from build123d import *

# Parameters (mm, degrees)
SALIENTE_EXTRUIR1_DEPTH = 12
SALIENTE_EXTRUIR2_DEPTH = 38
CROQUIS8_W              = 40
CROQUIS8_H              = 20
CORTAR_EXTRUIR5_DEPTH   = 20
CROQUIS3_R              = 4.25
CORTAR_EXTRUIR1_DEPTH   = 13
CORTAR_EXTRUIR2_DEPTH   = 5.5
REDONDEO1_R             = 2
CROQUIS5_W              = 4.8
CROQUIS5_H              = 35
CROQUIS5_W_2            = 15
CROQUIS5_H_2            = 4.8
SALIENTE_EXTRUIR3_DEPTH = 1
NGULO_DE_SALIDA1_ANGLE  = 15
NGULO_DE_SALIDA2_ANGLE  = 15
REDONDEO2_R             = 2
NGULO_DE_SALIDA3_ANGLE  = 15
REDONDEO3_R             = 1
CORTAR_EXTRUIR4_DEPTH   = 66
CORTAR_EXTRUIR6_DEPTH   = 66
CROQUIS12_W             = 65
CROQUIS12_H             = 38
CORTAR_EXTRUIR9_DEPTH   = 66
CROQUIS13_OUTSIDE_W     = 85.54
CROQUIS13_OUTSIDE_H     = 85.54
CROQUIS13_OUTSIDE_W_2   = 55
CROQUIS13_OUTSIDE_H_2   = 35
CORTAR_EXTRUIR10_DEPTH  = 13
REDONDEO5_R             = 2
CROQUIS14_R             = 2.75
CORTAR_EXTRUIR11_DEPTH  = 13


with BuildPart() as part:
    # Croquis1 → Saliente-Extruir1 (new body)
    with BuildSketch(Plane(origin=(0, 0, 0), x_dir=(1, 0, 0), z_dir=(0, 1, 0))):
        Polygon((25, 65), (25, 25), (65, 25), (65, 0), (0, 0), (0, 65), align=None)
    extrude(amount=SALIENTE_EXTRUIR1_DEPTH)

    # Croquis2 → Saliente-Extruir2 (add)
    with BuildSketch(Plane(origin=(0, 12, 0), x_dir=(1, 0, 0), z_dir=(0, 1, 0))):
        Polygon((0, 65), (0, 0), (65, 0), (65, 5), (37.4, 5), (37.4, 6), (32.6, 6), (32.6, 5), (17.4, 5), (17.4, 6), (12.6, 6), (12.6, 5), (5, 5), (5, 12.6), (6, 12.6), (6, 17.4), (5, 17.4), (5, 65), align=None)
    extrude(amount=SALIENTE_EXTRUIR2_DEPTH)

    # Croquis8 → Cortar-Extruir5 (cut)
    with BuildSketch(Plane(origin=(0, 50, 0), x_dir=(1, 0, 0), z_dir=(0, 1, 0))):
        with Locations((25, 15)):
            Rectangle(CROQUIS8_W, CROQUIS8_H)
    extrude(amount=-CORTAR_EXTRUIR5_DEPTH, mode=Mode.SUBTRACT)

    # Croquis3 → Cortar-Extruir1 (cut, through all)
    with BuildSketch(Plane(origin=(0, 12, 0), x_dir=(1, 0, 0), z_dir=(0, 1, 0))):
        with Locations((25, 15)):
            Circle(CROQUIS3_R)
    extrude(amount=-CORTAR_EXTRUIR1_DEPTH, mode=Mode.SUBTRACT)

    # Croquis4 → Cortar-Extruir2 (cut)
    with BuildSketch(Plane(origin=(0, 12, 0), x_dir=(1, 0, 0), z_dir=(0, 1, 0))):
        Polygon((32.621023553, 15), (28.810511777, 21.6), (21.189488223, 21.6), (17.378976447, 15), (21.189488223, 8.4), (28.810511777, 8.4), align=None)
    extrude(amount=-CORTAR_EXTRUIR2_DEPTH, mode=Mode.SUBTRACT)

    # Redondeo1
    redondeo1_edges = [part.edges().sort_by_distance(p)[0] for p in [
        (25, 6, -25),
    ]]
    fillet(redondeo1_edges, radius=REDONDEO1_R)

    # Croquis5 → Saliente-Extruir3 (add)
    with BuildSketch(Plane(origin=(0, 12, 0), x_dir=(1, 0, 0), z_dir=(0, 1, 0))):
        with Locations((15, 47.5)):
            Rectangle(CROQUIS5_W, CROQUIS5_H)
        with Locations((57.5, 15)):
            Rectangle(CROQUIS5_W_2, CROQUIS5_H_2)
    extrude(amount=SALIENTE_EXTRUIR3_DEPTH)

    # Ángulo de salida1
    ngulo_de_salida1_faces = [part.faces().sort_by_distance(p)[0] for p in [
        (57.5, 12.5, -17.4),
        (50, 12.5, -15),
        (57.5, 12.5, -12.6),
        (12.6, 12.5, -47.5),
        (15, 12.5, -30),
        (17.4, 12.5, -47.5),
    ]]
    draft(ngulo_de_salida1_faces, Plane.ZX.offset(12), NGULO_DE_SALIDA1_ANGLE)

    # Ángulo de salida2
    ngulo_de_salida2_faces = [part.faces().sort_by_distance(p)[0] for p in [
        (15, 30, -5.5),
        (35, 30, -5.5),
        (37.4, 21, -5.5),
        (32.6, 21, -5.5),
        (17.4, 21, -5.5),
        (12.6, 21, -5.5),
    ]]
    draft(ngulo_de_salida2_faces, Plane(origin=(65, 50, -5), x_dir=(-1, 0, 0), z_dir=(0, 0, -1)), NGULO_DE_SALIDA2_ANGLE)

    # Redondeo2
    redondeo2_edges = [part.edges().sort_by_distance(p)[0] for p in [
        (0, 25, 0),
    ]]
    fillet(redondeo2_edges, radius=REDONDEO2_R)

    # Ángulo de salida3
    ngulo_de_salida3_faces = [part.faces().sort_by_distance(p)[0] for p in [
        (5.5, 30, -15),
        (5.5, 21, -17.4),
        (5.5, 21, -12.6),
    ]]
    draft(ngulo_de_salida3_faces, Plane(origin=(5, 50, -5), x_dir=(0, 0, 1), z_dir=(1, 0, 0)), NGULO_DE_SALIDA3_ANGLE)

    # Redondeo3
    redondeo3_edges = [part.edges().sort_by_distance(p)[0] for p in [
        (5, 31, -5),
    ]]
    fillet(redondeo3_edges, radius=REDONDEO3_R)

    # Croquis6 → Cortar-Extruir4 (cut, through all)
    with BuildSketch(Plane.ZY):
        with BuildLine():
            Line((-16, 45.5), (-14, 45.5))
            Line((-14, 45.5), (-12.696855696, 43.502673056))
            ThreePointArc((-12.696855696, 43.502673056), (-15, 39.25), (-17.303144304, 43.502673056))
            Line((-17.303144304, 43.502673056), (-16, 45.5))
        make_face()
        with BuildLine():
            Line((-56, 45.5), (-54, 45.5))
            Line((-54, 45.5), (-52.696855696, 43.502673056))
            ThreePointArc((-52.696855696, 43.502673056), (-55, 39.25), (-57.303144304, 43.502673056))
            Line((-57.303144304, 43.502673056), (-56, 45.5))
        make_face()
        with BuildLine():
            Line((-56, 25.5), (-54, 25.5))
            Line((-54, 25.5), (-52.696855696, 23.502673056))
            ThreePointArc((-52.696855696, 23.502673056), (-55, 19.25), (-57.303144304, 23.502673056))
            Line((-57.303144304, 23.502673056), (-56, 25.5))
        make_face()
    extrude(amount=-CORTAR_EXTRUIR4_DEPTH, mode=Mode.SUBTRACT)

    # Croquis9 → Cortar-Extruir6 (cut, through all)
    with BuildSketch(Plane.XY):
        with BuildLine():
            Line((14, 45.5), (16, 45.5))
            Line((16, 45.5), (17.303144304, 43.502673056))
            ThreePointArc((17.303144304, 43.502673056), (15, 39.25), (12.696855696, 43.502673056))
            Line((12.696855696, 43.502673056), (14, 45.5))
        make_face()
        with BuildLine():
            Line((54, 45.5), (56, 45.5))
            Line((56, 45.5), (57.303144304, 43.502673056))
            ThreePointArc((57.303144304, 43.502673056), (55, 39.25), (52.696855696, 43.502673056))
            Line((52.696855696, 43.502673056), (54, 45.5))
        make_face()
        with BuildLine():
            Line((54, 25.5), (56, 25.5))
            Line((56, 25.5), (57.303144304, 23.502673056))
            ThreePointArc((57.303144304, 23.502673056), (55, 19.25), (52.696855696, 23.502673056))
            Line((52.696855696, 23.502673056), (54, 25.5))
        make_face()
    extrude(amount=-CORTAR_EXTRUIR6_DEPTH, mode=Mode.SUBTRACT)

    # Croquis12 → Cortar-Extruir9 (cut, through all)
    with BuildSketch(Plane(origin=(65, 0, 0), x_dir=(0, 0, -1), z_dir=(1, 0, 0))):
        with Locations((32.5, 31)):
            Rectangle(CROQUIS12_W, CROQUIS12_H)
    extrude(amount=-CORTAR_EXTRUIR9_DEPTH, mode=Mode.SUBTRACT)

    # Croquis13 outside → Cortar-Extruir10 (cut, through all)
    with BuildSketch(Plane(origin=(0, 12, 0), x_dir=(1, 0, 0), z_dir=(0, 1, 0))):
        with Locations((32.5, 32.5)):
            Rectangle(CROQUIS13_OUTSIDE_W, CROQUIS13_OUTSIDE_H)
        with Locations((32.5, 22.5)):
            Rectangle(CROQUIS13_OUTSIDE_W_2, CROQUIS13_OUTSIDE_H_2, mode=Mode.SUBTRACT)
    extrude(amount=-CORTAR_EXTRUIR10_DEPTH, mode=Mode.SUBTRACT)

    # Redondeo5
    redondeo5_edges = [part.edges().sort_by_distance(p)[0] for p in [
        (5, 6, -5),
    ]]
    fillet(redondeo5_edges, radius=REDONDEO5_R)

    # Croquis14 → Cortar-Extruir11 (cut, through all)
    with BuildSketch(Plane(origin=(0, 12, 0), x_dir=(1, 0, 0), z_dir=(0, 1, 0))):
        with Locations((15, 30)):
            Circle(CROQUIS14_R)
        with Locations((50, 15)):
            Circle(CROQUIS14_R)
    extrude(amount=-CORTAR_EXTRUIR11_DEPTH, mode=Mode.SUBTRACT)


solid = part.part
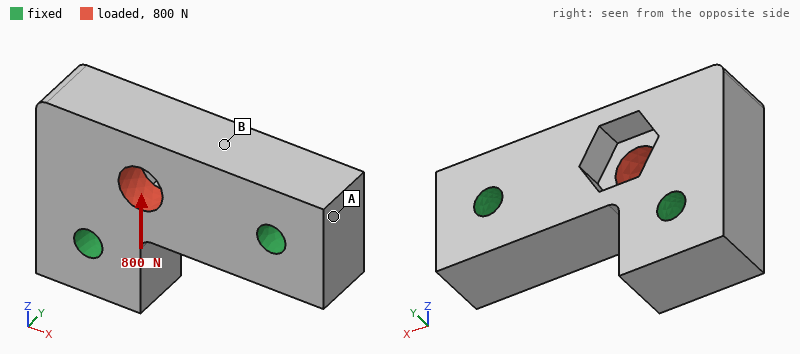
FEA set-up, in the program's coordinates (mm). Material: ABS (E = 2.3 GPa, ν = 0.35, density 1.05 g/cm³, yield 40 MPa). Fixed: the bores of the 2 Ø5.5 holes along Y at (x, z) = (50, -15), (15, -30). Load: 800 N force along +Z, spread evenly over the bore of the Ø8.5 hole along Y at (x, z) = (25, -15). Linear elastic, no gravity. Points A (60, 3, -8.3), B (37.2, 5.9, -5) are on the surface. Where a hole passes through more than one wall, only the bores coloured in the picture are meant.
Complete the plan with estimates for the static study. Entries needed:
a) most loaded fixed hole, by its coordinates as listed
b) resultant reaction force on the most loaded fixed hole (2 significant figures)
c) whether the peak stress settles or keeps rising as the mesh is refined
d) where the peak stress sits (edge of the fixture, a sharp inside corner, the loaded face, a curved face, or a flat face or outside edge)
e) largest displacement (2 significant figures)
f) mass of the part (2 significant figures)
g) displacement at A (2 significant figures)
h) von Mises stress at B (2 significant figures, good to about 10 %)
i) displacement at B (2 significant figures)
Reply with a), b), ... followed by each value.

a) (15, -30)
b) 630 N
c) keeps rising
d) edge of the fixture
e) 88 µm
f) 16 g
g) 14 µm
h) 2.4 MPa
i) 42 µm
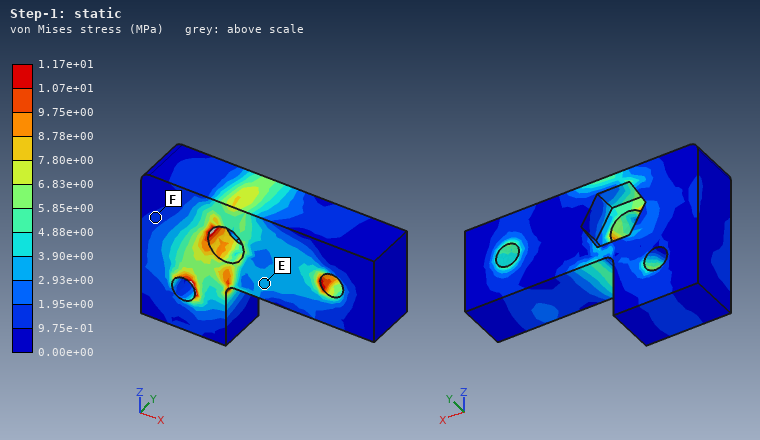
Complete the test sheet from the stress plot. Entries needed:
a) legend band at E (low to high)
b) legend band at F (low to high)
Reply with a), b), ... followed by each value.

a) 2.93e+00 to 3.90e+00 MPa
b) 9.75e-01 to 1.95e+00 MPa
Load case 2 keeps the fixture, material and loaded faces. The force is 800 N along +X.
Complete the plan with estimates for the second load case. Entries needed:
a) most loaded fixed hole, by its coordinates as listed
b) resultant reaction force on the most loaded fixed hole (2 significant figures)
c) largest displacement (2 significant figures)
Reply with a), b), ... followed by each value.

a) (50, -15)
b) 540 N
c) 61 µm
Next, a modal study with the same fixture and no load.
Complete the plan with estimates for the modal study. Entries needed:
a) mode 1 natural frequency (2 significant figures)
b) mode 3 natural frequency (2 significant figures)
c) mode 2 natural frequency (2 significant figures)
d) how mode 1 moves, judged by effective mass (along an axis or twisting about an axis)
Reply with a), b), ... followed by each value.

a) 4400 Hz
b) 8200 Hz
c) 7700 Hz
d) along Y
